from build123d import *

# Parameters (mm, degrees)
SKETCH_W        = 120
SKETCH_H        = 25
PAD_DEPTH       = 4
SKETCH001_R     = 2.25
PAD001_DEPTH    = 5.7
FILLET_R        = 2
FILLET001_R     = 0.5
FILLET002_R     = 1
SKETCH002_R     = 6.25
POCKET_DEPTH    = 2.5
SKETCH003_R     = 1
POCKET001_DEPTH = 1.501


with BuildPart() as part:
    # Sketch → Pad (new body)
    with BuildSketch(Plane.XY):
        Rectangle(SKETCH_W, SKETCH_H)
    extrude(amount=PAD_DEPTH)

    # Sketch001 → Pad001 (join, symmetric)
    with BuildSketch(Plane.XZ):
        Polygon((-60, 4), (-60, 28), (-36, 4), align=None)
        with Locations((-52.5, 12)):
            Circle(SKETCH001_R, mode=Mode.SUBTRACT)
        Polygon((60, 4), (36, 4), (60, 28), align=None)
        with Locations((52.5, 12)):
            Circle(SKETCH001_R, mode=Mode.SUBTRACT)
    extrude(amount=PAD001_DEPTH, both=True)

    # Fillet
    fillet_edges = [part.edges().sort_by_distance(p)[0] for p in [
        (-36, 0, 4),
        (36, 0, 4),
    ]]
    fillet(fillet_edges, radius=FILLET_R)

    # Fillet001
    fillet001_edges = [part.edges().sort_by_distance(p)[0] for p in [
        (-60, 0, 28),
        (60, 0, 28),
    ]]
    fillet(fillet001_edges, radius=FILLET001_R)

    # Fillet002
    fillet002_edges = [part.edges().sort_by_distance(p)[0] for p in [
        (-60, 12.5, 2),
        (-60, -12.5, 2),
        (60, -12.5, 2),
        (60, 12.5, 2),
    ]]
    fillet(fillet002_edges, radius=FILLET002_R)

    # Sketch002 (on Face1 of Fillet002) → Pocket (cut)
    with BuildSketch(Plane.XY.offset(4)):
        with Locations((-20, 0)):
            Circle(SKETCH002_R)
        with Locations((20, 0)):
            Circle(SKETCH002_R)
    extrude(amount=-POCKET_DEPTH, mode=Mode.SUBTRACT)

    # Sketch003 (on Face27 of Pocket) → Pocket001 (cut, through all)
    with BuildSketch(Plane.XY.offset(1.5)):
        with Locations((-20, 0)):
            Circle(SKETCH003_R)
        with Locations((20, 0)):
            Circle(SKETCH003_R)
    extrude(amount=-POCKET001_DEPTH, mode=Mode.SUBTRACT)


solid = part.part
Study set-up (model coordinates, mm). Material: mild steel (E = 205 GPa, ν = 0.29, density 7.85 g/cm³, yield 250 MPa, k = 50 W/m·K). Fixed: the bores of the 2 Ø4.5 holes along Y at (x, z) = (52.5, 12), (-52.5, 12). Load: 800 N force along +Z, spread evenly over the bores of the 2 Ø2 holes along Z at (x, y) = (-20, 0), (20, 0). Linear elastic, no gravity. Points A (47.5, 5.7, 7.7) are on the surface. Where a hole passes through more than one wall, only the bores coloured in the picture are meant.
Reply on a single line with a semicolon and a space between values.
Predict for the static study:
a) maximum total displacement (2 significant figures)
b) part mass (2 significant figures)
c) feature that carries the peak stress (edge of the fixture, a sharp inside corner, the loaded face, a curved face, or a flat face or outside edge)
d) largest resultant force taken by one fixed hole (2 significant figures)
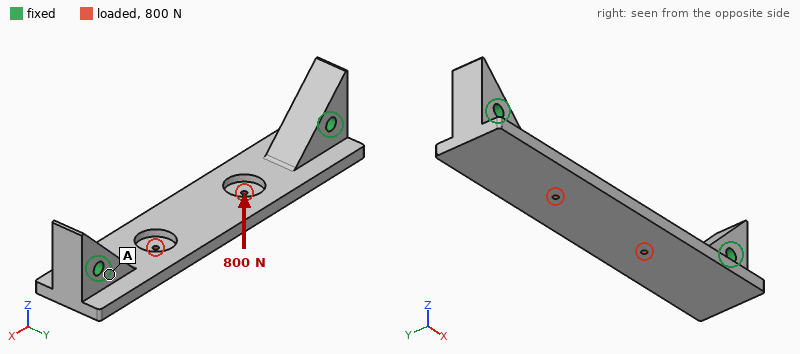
45 µm; 140 g; the loaded face; 770 N
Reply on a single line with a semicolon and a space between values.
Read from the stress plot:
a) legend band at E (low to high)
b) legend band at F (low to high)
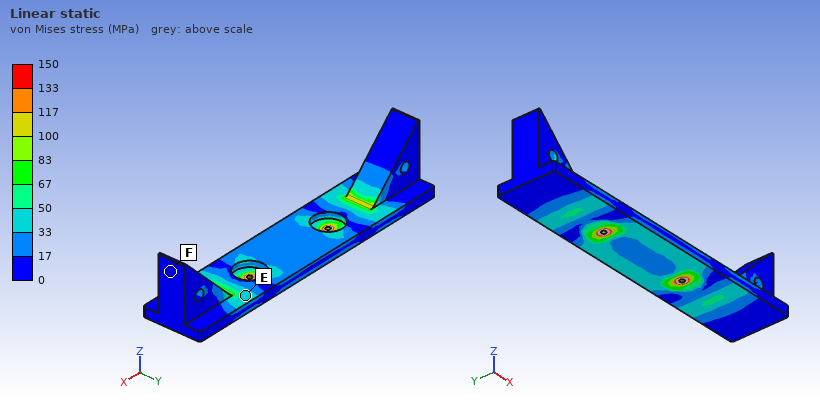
33 to 50 MPa; 0 to 17 MPa
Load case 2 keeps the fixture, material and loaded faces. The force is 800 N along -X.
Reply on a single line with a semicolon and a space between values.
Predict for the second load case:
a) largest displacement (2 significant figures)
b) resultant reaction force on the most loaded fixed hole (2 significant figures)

3.0 µm; 400 N
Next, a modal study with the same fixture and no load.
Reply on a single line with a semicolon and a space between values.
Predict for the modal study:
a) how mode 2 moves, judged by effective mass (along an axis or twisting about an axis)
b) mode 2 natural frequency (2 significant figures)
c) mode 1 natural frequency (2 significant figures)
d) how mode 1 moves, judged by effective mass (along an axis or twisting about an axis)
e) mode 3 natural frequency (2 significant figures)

twisting about X; 5800 Hz; 3100 Hz; along Z; 7100 Hz
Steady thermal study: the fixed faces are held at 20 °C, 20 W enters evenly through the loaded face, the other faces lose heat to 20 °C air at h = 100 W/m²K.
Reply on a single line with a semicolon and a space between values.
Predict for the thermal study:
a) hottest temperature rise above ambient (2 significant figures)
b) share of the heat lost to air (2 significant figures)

67 K; 61 %
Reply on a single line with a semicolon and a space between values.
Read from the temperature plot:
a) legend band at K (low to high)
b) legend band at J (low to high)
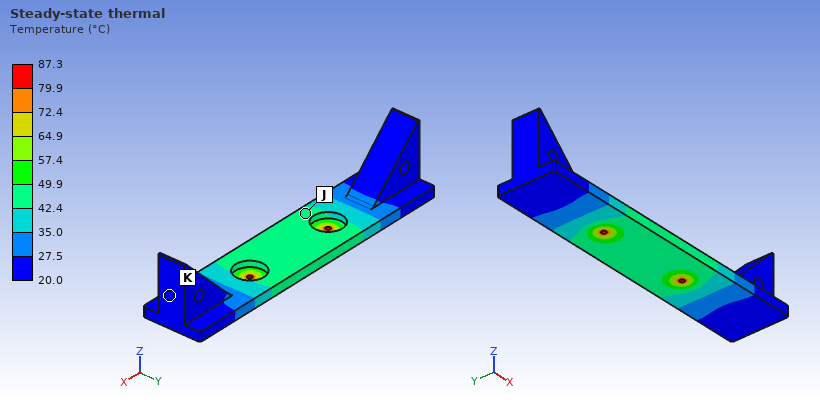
20.0 to 27.5 °C; 42.4 to 49.9 °C
